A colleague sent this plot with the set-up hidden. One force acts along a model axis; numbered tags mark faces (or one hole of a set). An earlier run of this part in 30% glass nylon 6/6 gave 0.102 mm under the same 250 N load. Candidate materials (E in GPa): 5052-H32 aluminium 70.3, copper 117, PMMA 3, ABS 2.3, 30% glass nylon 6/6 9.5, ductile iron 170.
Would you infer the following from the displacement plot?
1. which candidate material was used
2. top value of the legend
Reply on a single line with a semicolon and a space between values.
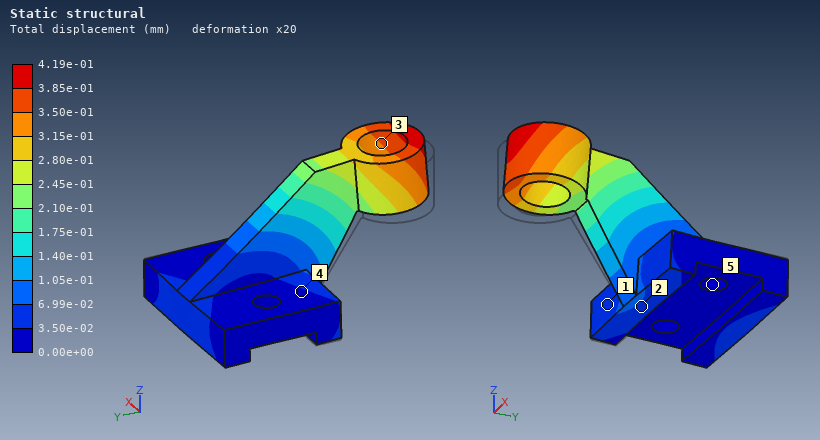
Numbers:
ABS; 4.19e-01 mm
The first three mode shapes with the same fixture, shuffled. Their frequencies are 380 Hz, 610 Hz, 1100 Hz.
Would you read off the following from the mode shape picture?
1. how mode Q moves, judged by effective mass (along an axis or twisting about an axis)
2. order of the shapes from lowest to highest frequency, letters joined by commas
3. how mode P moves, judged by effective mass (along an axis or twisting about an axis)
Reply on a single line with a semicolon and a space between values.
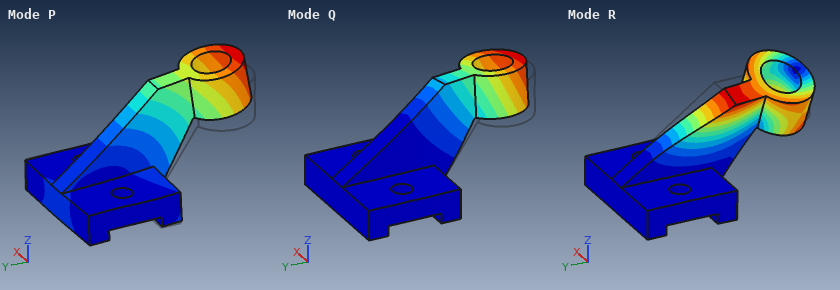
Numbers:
along X; Q, P, R; along Z
